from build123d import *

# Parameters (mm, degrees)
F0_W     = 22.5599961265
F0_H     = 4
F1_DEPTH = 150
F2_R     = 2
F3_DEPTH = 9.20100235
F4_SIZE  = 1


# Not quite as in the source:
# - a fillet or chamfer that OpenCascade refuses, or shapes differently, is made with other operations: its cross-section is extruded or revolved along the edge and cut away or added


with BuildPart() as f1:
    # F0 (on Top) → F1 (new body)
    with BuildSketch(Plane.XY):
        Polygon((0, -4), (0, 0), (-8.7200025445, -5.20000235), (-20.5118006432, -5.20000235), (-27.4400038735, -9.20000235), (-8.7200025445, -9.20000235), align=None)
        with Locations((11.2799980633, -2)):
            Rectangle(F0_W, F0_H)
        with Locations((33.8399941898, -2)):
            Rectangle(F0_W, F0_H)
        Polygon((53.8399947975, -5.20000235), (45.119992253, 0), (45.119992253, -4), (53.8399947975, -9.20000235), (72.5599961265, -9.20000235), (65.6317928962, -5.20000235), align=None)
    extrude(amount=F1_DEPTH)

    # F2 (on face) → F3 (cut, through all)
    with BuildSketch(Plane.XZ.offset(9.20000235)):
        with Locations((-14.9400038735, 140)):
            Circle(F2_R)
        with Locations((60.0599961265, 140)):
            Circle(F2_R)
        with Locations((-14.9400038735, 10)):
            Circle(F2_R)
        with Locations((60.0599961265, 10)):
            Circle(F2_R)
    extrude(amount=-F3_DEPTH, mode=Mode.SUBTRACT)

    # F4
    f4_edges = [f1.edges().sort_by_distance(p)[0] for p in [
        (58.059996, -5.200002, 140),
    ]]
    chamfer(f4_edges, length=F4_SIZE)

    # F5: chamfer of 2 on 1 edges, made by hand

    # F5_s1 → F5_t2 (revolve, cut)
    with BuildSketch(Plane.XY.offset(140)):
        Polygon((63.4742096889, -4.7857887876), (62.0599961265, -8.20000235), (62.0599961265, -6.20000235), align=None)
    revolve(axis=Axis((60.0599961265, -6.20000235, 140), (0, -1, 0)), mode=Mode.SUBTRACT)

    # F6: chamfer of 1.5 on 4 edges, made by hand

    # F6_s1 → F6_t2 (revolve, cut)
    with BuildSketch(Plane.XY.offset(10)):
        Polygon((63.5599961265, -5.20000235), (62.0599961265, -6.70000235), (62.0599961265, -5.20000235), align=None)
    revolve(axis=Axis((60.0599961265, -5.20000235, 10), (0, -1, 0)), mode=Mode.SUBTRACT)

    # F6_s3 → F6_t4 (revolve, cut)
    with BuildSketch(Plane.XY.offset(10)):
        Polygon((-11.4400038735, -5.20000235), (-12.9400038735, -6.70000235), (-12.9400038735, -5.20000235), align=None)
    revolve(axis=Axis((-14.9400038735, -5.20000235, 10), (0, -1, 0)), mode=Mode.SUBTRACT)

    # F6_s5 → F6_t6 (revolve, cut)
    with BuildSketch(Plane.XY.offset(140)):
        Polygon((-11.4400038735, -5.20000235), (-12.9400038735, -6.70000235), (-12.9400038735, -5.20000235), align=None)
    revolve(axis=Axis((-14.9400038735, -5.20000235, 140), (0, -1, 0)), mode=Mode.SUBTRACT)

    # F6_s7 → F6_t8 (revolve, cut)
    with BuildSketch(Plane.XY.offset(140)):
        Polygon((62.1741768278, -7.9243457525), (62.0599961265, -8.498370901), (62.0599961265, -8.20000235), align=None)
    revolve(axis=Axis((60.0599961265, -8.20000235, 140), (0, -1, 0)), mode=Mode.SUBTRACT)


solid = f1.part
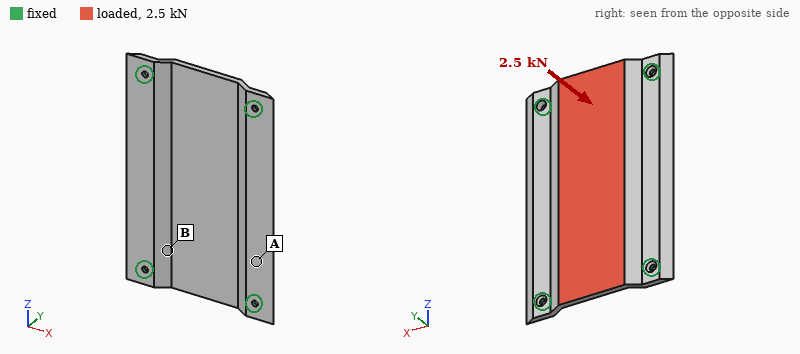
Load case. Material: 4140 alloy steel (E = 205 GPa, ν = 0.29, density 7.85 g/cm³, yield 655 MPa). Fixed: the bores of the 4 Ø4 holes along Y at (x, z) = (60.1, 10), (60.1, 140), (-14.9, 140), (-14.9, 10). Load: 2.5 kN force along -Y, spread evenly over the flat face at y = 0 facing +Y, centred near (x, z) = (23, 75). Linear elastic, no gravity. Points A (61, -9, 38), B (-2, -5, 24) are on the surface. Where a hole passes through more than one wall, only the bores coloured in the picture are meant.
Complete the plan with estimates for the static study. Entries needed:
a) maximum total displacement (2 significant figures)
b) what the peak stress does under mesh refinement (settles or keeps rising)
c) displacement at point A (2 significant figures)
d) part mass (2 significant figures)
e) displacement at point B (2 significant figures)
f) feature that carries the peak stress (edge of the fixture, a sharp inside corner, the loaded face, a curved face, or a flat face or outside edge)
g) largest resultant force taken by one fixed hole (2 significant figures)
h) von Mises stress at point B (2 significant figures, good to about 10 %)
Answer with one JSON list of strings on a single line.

["79 µm", "keeps rising", "33 µm", "440 g", "22 µm", "edge of the fixture", "2.3 kN", "35 MPa"]
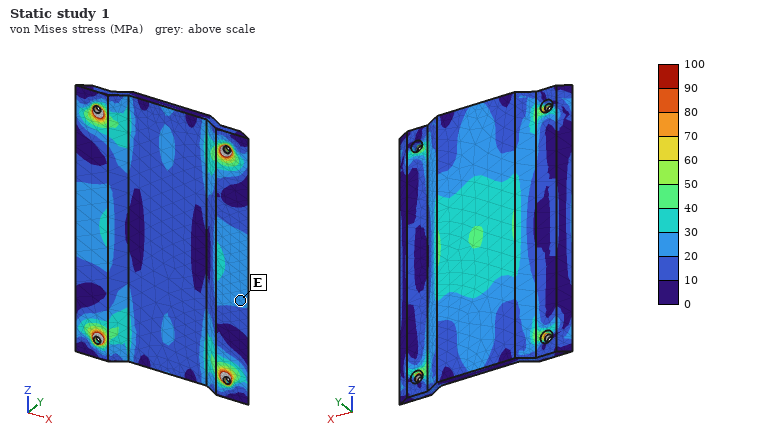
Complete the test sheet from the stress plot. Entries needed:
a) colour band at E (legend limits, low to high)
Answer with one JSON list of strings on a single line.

["20 to 30 MPa"]
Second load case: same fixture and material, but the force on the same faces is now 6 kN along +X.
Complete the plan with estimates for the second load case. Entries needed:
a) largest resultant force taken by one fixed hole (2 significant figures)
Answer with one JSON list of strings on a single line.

["1.8 kN"]
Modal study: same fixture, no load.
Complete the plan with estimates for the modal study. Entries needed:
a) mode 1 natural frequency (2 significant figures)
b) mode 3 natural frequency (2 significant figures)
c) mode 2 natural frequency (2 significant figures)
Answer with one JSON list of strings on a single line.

["1600 Hz", "3300 Hz", "1600 Hz"]
